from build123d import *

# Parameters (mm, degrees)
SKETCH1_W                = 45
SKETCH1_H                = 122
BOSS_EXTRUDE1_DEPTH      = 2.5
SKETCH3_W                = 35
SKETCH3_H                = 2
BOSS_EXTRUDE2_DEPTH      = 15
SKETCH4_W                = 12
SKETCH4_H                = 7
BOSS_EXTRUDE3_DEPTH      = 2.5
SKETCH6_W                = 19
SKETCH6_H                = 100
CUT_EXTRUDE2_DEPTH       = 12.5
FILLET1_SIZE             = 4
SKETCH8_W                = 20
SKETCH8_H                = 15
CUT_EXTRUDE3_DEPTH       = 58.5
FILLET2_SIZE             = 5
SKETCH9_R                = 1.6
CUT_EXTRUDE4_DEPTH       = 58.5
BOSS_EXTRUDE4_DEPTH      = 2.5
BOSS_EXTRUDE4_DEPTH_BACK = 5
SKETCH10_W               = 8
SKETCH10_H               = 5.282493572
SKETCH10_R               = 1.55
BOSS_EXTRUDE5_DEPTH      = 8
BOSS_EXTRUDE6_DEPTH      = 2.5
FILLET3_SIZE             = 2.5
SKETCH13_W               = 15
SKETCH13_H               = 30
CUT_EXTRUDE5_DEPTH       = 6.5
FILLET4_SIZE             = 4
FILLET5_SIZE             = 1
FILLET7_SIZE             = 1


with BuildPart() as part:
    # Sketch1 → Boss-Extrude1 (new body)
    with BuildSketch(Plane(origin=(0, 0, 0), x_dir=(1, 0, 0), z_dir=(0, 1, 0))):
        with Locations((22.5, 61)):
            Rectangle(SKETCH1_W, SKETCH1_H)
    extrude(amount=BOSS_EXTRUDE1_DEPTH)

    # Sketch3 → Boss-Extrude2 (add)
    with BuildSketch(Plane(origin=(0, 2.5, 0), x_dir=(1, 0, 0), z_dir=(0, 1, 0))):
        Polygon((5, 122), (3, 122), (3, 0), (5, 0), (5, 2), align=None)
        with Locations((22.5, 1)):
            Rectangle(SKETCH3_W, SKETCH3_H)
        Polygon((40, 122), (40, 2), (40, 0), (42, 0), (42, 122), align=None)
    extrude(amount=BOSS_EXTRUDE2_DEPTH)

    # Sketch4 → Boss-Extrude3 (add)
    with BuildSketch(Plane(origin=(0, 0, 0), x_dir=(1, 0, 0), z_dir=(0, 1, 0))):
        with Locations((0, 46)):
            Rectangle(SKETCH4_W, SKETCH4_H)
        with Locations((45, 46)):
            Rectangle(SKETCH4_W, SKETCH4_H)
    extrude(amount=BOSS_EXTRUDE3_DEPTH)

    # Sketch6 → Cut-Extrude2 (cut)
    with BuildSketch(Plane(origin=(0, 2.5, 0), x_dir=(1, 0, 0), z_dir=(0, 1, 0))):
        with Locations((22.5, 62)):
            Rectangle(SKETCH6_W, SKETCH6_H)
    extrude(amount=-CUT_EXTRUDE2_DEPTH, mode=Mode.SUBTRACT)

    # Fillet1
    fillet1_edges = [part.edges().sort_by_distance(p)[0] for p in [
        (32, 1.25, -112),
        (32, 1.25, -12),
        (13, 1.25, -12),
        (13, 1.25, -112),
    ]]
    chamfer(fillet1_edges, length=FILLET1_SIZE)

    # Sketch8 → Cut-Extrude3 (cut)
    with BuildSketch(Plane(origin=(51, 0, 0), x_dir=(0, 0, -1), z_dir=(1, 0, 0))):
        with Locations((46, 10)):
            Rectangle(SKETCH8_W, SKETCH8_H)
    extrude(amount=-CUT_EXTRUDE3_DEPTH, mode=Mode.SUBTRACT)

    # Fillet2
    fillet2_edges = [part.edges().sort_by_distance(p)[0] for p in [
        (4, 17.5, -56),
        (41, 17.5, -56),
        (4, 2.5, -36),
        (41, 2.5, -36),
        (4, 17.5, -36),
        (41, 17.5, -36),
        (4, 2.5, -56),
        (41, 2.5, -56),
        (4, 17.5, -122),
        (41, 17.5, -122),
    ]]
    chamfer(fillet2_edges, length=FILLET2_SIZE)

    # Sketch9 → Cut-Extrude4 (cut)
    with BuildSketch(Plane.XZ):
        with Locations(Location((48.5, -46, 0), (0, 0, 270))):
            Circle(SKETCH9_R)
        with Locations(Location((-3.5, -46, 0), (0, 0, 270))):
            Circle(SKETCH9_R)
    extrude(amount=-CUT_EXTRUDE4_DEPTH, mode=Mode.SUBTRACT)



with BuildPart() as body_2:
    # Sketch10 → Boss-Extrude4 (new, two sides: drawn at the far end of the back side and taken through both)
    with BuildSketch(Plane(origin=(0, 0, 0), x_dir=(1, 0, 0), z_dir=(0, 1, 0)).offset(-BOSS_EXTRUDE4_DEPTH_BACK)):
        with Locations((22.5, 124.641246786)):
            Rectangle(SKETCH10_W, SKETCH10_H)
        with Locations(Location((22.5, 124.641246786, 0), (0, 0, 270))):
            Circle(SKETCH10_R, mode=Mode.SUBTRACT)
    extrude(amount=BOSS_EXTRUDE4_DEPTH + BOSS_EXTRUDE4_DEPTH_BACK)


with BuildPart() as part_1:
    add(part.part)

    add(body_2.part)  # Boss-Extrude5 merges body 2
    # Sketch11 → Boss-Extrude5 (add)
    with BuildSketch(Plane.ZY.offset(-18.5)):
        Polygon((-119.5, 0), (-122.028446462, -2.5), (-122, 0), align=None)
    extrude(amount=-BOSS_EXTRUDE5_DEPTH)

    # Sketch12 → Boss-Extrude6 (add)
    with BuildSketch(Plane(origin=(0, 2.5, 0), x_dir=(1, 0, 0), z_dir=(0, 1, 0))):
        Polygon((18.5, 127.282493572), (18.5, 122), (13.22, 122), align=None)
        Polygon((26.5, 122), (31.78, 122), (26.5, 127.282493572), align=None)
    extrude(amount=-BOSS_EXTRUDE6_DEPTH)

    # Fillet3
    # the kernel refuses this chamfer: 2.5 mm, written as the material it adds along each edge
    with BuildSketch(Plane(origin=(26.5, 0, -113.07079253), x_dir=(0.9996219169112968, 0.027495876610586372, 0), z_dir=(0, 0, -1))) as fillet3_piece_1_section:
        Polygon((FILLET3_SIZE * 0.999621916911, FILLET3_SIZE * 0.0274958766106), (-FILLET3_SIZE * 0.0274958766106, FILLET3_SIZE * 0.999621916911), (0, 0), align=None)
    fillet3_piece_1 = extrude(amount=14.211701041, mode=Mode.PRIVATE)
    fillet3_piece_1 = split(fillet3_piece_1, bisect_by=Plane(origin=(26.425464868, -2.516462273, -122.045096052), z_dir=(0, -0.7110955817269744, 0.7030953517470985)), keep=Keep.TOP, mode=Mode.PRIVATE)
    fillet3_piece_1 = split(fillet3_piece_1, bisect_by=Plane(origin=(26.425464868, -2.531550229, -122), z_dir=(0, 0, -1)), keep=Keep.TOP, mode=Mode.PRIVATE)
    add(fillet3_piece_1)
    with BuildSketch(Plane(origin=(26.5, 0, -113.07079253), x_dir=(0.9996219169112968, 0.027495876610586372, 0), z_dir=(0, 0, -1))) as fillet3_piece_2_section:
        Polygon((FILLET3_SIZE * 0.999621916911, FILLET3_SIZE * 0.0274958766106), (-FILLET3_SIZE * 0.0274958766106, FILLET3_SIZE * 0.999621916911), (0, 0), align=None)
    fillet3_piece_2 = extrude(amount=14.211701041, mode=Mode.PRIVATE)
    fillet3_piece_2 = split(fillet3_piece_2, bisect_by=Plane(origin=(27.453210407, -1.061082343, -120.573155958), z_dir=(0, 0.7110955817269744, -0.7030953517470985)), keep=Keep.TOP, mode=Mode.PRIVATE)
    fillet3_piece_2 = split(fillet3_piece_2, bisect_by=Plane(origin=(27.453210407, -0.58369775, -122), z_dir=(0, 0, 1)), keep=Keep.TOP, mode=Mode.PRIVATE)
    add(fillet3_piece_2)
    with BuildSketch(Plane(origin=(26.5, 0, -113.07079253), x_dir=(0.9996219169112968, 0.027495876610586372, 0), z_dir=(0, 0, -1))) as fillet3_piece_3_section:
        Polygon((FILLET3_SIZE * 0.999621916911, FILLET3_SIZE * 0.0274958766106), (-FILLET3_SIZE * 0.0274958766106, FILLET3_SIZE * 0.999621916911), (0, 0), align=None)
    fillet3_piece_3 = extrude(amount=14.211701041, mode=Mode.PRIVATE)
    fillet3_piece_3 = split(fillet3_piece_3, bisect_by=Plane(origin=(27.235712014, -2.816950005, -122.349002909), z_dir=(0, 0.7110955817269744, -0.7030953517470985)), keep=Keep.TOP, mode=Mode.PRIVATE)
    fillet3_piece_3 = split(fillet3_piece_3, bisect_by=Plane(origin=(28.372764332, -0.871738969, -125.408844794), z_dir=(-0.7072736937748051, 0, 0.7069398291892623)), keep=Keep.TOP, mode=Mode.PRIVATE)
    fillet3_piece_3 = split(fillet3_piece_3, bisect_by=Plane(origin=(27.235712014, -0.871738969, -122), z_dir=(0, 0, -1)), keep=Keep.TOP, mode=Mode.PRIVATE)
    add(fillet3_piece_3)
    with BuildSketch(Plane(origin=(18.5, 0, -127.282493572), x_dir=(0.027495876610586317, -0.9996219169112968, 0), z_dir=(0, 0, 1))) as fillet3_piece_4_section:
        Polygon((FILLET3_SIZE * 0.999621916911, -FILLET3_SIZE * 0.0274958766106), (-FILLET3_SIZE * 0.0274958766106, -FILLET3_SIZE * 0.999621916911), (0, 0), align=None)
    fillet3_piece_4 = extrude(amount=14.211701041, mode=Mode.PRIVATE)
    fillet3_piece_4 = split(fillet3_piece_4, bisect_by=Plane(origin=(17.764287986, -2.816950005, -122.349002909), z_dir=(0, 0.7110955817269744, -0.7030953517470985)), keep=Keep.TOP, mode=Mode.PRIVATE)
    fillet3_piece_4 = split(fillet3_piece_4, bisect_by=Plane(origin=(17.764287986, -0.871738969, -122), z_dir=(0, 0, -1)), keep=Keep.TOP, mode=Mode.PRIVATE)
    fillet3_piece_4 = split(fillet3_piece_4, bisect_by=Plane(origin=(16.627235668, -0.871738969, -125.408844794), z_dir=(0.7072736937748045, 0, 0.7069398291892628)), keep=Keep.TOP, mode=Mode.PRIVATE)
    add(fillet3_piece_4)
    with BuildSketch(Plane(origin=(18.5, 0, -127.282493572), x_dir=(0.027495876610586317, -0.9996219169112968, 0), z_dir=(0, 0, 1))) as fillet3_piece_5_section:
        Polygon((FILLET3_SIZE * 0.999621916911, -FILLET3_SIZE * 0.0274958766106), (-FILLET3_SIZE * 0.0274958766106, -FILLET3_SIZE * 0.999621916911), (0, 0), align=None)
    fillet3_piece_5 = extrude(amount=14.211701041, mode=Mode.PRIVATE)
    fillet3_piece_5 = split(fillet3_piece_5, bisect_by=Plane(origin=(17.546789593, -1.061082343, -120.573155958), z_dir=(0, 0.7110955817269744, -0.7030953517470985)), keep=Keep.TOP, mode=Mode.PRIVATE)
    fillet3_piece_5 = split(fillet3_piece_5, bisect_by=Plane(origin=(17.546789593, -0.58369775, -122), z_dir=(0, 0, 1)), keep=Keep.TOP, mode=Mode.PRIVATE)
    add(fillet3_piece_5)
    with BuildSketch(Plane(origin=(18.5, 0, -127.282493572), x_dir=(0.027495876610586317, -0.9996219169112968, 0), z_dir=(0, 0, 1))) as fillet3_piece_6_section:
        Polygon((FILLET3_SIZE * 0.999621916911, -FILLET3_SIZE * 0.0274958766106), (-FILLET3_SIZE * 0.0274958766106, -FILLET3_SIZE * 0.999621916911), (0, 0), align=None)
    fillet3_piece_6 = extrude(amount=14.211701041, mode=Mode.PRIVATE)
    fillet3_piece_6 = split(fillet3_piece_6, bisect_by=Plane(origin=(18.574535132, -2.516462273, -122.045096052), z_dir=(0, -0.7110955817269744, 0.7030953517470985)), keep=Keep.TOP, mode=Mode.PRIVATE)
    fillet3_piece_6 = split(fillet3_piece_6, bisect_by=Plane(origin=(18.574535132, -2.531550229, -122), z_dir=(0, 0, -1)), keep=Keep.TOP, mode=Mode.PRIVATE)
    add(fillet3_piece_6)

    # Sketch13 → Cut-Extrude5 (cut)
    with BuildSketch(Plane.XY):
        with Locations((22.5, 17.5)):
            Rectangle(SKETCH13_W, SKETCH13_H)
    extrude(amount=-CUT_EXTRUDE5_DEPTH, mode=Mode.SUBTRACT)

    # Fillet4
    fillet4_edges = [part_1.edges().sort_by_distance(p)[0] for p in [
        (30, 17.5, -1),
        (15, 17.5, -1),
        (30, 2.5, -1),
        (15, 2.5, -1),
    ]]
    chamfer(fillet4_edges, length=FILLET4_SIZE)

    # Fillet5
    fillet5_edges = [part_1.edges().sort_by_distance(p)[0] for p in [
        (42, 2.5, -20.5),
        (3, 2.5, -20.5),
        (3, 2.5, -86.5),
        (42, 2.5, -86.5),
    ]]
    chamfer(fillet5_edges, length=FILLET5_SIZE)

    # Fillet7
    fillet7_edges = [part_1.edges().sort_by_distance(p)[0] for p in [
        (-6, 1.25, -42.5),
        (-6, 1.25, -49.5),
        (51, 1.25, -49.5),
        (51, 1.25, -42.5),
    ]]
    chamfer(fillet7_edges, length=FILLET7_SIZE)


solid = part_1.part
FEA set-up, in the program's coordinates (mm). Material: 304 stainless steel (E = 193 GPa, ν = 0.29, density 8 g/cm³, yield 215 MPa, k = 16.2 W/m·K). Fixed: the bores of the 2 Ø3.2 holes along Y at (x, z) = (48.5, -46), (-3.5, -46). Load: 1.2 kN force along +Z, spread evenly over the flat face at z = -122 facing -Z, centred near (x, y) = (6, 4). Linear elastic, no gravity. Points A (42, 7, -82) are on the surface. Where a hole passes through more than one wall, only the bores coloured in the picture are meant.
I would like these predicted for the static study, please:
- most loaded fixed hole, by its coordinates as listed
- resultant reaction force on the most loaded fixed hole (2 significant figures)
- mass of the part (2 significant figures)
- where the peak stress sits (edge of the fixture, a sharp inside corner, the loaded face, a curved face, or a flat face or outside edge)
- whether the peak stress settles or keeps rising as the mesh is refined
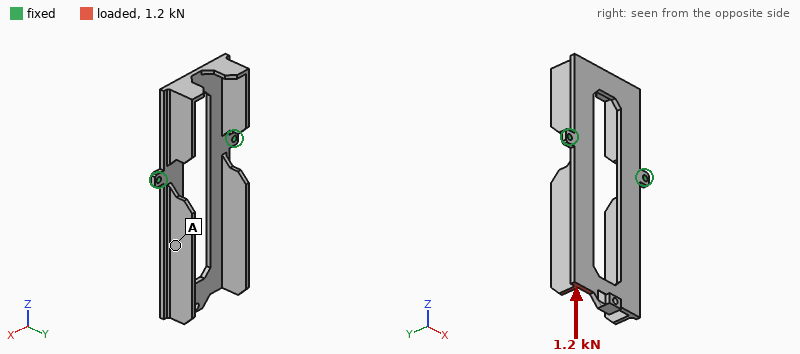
(-3.5, -46)
1.1 kN
130 g
edge of the fixture
keeps rising
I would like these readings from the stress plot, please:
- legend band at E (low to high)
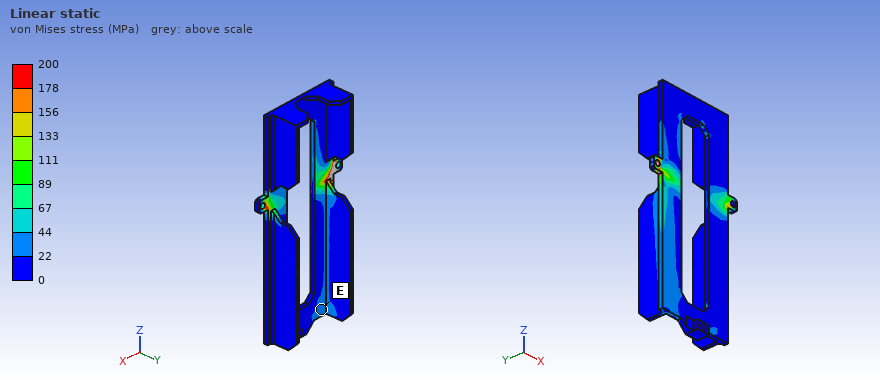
22 to 44 MPa
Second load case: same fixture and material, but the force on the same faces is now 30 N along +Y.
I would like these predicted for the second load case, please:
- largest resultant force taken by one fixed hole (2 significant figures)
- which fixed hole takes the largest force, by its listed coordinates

23 N
(-3.5, -46)
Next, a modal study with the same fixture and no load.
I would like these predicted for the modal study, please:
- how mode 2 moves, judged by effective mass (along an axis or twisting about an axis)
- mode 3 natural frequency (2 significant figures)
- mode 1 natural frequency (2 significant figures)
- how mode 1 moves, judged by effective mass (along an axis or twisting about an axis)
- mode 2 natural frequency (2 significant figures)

along Y
790 Hz
250 Hz
along Y
590 Hz
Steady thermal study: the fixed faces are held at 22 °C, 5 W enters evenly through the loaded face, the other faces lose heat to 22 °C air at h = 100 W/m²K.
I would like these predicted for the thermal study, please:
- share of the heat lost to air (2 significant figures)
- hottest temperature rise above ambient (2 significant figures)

100 %
62 K
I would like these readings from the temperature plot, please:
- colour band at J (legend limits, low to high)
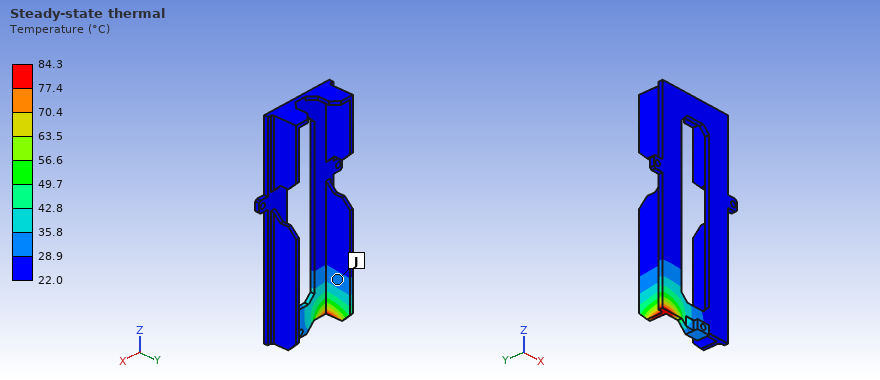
28.9 to 35.8 °C
